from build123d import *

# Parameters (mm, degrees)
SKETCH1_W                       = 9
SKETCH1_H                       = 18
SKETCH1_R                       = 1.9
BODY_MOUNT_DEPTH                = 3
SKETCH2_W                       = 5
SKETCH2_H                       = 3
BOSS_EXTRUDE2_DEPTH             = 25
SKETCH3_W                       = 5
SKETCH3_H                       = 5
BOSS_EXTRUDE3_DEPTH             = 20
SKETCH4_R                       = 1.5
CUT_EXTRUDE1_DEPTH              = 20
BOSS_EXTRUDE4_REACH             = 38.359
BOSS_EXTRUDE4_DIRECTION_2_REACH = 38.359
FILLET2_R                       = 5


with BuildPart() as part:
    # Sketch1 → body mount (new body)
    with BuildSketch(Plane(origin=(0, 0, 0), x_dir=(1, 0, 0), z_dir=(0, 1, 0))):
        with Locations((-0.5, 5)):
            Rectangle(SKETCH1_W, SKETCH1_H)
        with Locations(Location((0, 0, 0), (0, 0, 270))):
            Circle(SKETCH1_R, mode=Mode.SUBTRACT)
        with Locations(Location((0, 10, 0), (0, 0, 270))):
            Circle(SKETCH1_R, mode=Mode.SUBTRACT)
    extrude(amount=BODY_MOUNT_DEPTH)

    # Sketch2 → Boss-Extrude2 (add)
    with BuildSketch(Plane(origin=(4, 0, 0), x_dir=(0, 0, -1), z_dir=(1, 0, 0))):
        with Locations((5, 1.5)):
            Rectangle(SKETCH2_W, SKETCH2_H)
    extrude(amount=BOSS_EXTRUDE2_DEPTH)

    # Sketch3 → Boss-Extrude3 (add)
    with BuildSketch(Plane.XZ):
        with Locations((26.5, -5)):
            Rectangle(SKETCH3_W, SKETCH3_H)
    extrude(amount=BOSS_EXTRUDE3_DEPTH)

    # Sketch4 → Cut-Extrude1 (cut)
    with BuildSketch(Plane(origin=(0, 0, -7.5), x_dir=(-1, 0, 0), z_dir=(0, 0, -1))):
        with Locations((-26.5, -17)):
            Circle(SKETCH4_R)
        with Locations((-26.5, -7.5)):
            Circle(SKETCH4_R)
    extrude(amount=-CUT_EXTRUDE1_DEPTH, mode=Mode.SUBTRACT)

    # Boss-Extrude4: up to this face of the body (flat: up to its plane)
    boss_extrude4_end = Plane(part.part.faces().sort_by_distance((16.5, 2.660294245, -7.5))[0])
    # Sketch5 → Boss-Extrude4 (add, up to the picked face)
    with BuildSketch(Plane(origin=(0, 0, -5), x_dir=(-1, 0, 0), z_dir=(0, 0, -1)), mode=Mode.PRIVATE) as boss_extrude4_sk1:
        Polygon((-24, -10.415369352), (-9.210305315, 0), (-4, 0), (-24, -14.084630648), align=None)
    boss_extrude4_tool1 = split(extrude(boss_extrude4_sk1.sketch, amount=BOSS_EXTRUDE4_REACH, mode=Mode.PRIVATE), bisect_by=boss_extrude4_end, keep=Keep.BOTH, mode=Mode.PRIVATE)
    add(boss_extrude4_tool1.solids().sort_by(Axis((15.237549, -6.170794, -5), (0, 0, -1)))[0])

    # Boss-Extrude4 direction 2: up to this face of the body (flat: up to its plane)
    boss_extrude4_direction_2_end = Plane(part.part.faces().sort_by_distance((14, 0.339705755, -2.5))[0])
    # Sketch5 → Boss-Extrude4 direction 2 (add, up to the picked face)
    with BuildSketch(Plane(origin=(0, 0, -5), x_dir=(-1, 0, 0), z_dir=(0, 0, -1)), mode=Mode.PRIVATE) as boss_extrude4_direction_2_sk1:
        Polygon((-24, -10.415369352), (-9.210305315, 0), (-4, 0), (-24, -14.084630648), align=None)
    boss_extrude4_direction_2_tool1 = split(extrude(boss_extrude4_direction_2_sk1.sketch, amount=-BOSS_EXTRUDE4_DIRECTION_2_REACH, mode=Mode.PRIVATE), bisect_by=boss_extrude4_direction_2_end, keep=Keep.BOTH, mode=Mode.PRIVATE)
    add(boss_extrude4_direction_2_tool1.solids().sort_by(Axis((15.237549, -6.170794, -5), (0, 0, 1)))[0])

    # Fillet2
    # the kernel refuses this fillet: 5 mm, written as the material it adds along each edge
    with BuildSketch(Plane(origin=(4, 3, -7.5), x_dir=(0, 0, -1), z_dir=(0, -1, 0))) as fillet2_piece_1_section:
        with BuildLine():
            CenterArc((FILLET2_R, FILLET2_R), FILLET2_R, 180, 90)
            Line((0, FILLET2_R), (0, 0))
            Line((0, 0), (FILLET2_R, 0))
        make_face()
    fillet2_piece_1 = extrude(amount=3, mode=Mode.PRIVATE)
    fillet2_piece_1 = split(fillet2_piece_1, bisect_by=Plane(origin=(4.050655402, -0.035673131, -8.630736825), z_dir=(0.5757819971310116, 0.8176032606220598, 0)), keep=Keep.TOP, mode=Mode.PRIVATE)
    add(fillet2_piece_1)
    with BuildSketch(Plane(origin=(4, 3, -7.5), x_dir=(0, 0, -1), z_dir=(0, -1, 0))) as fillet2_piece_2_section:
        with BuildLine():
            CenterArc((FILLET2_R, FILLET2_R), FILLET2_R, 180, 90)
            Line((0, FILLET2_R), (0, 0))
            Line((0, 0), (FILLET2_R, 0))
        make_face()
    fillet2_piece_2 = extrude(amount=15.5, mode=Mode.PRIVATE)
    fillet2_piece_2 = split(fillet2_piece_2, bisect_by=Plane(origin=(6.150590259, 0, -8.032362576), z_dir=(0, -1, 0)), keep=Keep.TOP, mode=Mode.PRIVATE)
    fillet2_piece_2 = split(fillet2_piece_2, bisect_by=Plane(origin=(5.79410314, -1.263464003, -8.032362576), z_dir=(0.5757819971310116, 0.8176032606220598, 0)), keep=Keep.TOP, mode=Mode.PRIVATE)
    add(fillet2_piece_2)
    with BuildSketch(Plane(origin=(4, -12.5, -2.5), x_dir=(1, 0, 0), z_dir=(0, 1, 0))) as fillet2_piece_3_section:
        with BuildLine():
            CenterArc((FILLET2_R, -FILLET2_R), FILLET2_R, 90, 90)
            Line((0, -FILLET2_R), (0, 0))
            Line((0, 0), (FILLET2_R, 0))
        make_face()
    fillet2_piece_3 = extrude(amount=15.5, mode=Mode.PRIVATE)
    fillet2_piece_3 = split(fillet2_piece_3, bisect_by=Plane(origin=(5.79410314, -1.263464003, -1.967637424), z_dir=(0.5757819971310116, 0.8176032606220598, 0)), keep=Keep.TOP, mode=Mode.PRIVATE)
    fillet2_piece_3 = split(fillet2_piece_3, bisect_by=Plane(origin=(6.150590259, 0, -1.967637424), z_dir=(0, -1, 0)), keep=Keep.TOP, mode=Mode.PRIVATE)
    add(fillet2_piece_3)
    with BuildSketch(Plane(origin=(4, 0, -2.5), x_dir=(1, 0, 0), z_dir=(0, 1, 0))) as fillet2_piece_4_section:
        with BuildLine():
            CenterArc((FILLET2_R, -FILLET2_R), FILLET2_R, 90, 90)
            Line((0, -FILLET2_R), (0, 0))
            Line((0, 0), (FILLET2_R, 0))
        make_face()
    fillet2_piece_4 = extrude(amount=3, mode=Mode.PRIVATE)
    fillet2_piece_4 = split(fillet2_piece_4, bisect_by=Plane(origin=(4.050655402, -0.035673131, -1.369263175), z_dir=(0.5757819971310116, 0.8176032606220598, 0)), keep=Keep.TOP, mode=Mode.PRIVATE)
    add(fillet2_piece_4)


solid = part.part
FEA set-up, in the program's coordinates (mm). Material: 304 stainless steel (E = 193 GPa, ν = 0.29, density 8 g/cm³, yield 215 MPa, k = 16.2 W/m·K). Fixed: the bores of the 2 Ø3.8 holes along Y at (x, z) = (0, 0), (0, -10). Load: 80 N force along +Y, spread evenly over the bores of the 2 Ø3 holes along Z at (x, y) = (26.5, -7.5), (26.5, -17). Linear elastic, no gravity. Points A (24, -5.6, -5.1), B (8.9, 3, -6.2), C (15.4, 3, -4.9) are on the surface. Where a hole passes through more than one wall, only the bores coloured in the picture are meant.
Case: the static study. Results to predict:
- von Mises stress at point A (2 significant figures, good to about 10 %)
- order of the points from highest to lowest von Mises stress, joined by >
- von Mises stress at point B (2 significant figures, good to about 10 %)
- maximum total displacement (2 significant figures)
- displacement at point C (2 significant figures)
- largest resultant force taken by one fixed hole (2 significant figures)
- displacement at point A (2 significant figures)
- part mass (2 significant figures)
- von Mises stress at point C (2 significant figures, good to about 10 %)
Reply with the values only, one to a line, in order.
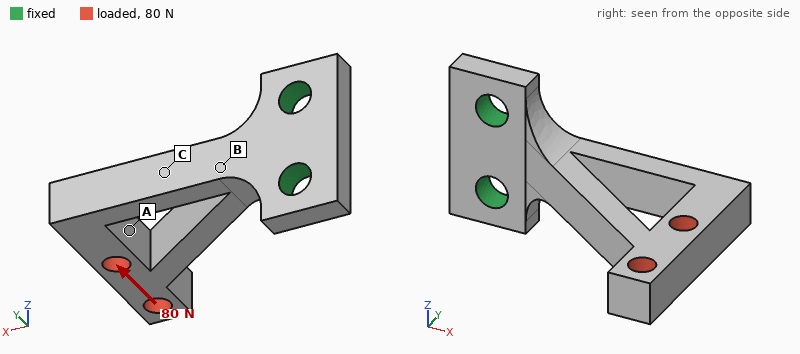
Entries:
16 MPa
B > C > A
75 MPa
0.12 mm
0.035 mm
40 N
0.074 mm
13 g
39 MPa
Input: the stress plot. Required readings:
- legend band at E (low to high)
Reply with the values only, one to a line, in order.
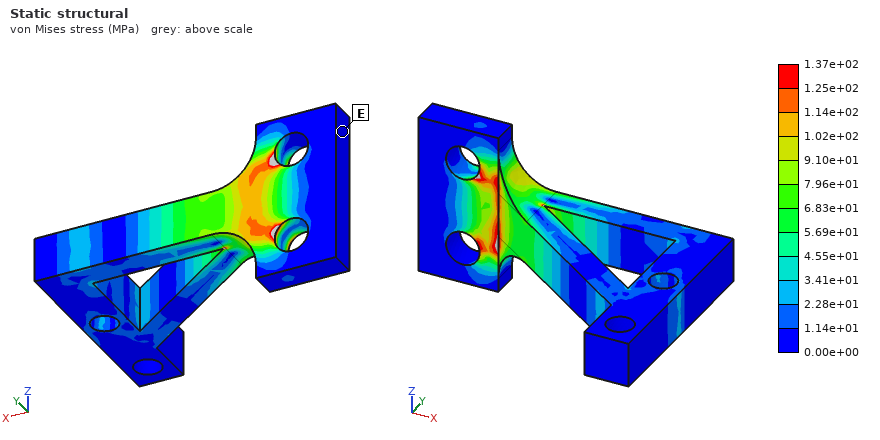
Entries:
0.00e+00 to 1.14e+01 MPa
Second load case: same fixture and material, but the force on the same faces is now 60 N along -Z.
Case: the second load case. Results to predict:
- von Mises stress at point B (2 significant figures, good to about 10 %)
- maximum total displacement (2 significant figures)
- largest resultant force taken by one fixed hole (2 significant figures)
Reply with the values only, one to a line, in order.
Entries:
22 MPa
52 µm
180 N
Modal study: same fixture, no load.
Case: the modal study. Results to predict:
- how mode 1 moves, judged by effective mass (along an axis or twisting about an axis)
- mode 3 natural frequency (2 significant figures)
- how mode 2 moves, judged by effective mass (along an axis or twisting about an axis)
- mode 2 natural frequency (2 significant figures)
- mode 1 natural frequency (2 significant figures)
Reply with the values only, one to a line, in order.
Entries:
along Y
6900 Hz
along Z
3400 Hz
2000 Hz
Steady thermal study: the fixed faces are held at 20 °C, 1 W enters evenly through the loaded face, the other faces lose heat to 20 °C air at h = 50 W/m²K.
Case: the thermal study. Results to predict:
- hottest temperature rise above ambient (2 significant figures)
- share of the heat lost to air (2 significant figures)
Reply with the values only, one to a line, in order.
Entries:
28 K
76 %
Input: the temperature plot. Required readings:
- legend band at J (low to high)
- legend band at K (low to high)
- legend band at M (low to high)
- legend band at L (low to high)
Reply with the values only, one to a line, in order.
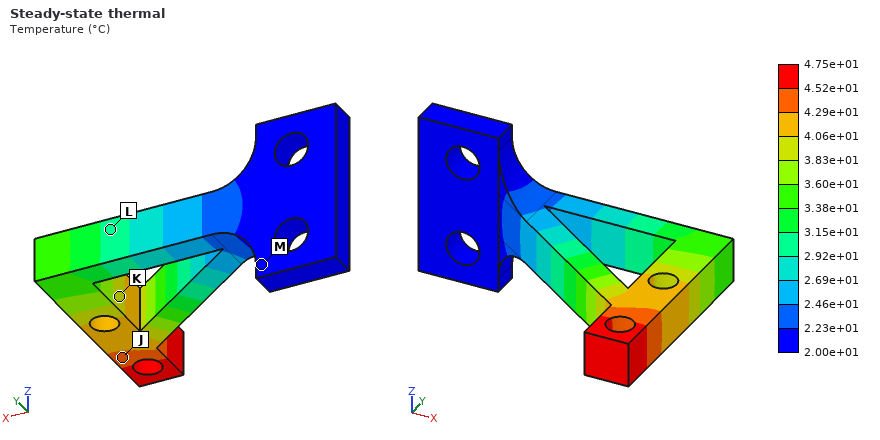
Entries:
4.29e+01 to 4.52e+01 °C
3.83e+01 to 4.06e+01 °C
2.00e+01 to 2.23e+01 °C
2.92e+01 to 3.15e+01 °C
